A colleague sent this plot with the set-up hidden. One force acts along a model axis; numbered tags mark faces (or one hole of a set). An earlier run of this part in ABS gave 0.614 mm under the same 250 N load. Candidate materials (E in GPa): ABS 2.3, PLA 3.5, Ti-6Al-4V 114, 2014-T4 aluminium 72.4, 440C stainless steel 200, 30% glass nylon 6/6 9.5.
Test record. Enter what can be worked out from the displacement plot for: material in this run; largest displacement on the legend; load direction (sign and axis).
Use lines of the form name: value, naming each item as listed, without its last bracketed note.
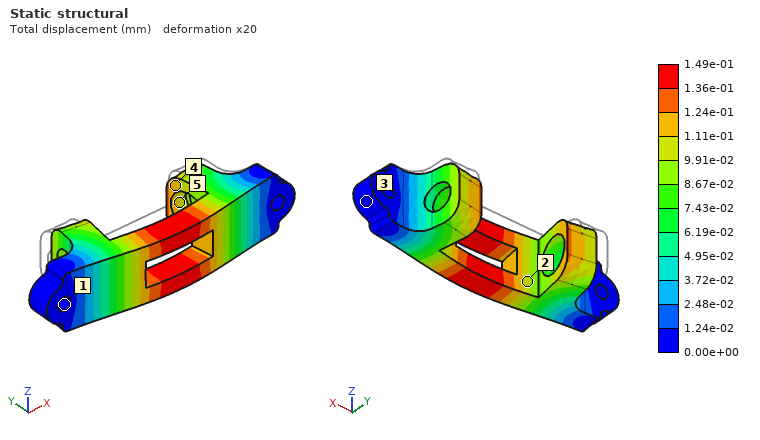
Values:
material in this run: 30% glass nylon 6/6
largest displacement on the legend: 1.49e-01 mm
load direction: -Y
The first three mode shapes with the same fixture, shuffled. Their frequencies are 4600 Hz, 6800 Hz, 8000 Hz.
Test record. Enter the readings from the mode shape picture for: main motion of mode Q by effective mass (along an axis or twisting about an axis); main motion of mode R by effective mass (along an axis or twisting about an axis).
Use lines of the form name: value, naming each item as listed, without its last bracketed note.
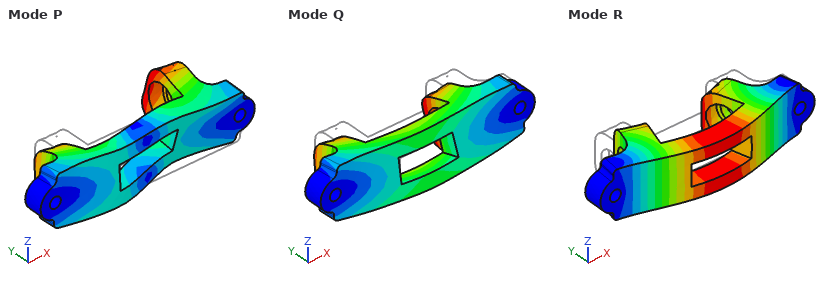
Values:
main motion of mode Q by effective mass: along Z
main motion of mode R by effective mass: along Y
